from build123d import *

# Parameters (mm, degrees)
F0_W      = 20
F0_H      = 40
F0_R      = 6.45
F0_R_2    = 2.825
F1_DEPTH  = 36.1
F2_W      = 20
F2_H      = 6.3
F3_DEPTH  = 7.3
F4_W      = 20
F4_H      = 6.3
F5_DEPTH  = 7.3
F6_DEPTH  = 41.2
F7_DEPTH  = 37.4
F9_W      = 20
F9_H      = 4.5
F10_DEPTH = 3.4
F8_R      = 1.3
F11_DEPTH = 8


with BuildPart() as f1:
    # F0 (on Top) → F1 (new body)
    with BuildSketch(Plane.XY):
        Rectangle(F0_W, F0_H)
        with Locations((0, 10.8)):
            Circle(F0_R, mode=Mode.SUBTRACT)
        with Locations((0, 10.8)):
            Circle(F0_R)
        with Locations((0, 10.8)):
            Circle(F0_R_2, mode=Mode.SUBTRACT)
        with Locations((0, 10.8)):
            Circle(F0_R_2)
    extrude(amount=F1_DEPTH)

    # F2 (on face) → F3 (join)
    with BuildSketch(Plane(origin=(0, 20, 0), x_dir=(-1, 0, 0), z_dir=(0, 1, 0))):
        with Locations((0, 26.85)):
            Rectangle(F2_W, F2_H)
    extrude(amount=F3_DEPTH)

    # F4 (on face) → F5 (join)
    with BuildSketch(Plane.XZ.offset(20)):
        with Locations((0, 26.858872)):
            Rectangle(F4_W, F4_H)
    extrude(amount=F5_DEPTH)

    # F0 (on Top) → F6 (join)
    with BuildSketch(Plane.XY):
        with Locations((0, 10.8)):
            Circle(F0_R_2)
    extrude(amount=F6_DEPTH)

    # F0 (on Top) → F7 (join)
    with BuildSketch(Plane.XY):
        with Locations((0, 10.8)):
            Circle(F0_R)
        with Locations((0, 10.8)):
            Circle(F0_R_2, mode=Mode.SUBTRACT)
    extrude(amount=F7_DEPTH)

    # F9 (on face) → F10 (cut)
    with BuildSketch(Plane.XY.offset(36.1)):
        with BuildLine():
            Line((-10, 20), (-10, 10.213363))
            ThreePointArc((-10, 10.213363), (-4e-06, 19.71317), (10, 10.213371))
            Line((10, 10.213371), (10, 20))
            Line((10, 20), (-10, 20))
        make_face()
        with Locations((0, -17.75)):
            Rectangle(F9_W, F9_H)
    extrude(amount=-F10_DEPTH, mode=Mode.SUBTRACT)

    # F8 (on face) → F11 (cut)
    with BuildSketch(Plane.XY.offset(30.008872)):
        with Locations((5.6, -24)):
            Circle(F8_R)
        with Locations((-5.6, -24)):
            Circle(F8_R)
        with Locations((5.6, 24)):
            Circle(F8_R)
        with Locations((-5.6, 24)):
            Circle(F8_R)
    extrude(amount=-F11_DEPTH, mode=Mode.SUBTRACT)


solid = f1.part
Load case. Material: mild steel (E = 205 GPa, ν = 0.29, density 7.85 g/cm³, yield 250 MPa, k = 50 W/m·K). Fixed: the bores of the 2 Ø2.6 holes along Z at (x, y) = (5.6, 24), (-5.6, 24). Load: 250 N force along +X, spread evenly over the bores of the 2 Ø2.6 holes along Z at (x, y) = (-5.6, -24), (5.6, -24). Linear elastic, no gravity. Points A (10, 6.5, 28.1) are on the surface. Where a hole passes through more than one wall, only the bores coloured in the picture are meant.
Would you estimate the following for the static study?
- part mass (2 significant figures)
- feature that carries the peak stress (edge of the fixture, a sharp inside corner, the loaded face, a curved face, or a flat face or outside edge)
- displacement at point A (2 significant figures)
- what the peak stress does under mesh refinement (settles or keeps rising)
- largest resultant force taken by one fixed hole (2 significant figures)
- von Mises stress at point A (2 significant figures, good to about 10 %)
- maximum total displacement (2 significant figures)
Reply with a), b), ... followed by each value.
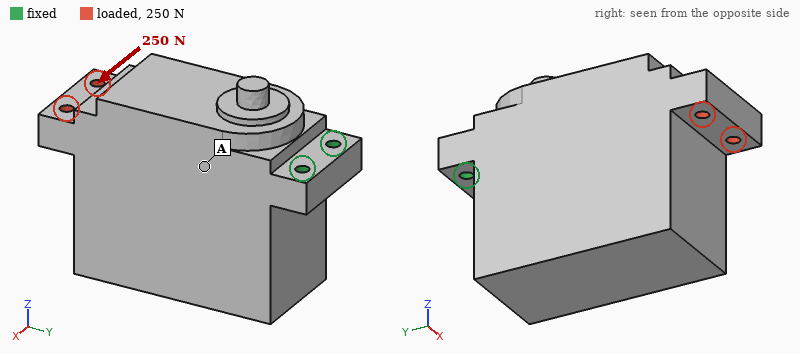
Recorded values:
a) 240 g
b) edge of the fixture
c) 2.7 µm
d) keeps rising
e) 950 N
f) 5.9 MPa
g) 8.9 µm
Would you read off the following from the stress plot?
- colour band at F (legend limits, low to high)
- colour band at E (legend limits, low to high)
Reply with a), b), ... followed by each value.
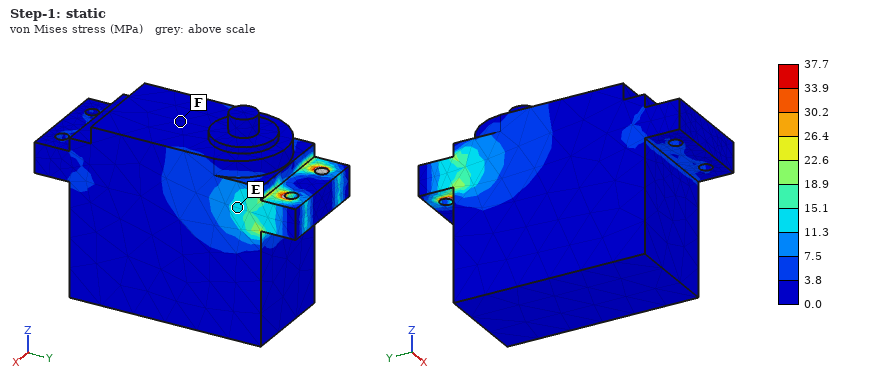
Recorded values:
a) 0.0 to 3.8 MPa
b) 11.3 to 15.1 MPa
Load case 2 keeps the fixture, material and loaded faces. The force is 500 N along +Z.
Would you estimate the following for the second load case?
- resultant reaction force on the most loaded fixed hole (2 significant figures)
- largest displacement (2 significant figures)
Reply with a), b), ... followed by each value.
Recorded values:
a) 250 N
b) 89 µm
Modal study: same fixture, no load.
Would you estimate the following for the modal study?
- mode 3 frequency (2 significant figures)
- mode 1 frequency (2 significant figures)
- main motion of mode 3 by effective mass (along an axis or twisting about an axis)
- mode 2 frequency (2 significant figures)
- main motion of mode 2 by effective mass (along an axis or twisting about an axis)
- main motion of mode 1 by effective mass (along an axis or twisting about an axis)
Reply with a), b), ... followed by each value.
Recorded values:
a) 5700 Hz
b) 1300 Hz
c) twisting about Y
d) 3200 Hz
e) along X
f) along Z
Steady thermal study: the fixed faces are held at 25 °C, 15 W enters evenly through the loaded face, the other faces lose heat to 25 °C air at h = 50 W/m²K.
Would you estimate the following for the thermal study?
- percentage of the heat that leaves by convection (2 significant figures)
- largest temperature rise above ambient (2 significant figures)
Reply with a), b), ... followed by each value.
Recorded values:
a) 38 %
b) 45 K
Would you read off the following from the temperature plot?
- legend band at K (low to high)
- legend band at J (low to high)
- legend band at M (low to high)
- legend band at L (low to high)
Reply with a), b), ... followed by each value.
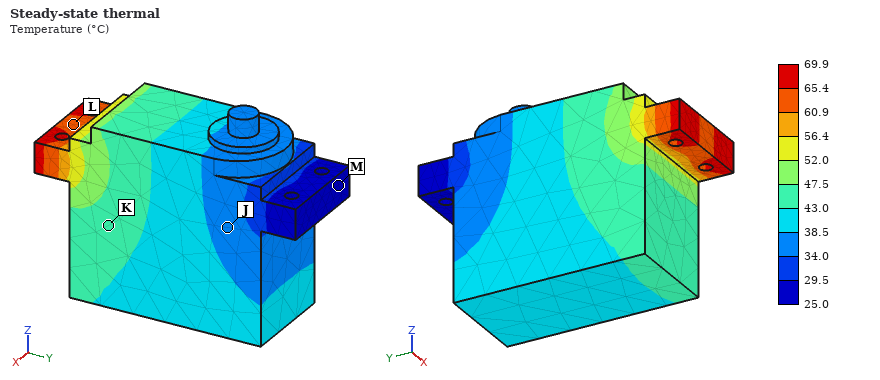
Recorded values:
a) 43.0 to 47.5 °C
b) 34.0 to 38.5 °C
c) 25.0 to 29.5 °C
d) 60.9 to 65.4 °C
